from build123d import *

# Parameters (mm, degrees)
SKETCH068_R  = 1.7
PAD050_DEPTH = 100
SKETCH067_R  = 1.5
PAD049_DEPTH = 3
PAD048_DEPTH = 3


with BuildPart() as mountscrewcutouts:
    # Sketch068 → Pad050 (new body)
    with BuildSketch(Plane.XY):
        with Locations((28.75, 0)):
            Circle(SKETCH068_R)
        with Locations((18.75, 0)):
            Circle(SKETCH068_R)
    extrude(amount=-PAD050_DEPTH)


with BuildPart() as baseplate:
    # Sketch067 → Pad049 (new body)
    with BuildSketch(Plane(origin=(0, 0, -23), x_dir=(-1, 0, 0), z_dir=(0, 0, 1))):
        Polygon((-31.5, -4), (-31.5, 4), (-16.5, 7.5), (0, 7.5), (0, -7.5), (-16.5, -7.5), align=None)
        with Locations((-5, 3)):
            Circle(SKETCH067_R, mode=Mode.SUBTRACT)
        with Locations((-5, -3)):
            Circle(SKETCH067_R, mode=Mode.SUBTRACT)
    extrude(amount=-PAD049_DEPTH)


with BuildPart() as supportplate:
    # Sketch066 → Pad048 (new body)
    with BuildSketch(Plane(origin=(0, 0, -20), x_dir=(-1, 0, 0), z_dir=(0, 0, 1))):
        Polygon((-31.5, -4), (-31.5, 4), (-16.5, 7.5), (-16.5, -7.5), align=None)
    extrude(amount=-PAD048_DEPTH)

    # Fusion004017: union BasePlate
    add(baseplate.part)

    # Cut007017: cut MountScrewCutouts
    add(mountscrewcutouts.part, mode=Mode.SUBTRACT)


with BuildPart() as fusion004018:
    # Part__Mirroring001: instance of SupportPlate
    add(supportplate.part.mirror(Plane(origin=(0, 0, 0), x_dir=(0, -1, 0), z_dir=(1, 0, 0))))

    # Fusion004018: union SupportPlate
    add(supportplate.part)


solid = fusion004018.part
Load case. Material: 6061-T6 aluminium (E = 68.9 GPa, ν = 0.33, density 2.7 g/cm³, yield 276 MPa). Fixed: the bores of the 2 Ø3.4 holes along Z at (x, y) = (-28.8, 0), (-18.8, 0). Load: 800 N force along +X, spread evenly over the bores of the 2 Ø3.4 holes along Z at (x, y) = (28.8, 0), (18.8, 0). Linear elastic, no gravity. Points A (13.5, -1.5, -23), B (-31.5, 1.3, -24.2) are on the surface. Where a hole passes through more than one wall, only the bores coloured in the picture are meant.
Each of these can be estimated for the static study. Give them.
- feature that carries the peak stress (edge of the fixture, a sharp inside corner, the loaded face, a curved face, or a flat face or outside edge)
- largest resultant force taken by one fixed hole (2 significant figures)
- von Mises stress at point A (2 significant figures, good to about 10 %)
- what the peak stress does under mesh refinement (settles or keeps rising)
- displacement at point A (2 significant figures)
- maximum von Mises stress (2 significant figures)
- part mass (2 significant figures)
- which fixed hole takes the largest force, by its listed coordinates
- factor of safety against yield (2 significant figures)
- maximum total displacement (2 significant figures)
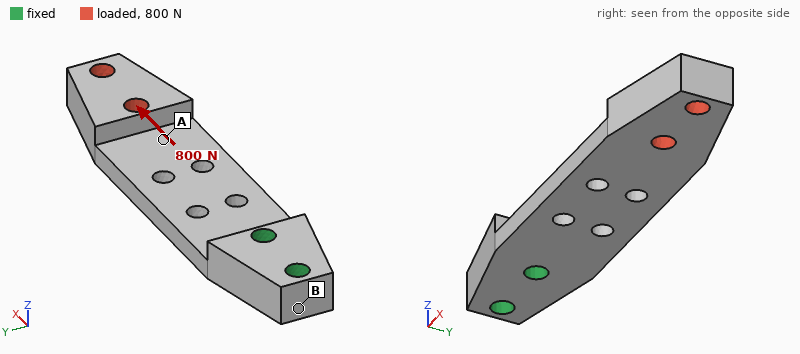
a curved face
640 N
67 MPa
settles
0.28 mm
190 MPa
8.8 g
(-18.8, 0)
1.4
0.65 mm
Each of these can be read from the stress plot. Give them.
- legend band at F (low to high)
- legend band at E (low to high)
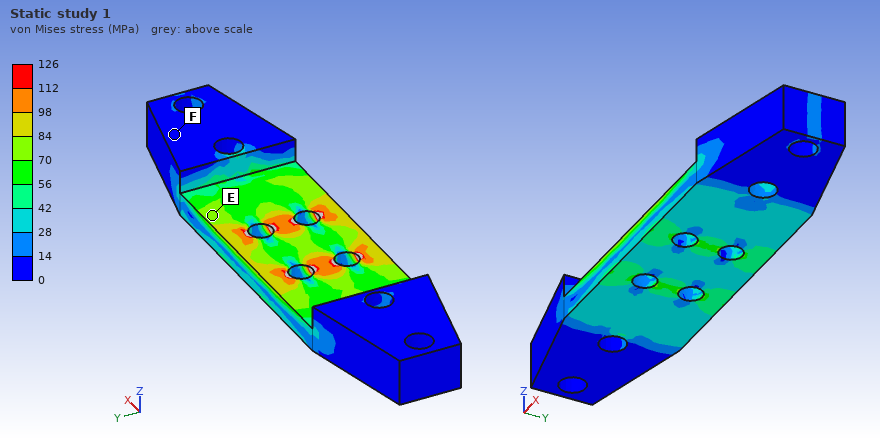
0 to 14 MPa
70 to 84 MPa
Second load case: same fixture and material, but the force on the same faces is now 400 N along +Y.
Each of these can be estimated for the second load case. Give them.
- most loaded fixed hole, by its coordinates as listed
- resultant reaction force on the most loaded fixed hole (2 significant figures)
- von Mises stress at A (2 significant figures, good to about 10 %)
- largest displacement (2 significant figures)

(-18.8, 0)
1.4 kN
39 MPa
0.37 mm
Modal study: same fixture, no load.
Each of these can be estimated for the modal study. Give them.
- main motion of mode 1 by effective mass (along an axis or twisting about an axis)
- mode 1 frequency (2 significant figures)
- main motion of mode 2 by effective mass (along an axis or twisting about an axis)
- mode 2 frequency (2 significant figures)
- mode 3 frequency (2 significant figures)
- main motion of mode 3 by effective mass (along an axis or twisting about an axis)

along Z
870 Hz
along Y
3400 Hz
5800 Hz
twisting about X
